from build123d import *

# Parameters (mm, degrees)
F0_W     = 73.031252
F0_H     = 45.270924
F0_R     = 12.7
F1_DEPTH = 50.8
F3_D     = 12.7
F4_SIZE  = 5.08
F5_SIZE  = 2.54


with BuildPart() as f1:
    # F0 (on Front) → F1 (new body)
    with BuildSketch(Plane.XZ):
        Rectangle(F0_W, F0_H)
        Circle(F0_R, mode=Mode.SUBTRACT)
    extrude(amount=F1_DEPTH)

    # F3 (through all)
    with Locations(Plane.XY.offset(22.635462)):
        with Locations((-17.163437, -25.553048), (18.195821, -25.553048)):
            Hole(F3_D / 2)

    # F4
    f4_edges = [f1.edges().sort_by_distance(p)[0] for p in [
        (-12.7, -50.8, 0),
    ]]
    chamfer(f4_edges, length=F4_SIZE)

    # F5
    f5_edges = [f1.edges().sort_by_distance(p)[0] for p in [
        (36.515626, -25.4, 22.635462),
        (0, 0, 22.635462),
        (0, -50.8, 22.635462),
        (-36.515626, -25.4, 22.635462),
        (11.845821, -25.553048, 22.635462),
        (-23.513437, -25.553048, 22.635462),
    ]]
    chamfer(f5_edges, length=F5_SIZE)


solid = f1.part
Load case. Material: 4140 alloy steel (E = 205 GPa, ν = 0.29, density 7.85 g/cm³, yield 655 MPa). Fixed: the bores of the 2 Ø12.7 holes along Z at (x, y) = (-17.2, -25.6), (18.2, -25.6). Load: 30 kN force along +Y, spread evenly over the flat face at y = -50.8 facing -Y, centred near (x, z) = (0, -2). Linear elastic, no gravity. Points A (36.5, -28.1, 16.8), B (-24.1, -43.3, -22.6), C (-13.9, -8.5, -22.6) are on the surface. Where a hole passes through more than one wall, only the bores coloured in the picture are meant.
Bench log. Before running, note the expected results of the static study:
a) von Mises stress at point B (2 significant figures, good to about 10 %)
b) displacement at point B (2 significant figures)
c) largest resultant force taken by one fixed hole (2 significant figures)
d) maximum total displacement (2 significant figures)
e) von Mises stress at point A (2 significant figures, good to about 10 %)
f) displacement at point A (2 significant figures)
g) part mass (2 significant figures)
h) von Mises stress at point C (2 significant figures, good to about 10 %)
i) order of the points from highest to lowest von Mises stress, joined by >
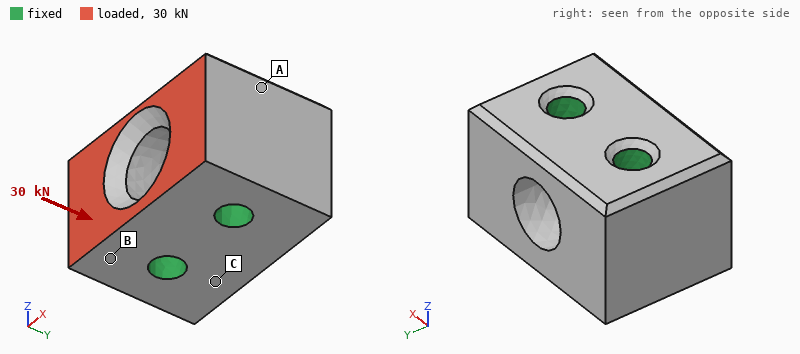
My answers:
16 MPa
1.7 µm
15 kN
3.2 µm
8.3 MPa
1.0 µm
1.0 kg
3.1 MPa
B > A > C
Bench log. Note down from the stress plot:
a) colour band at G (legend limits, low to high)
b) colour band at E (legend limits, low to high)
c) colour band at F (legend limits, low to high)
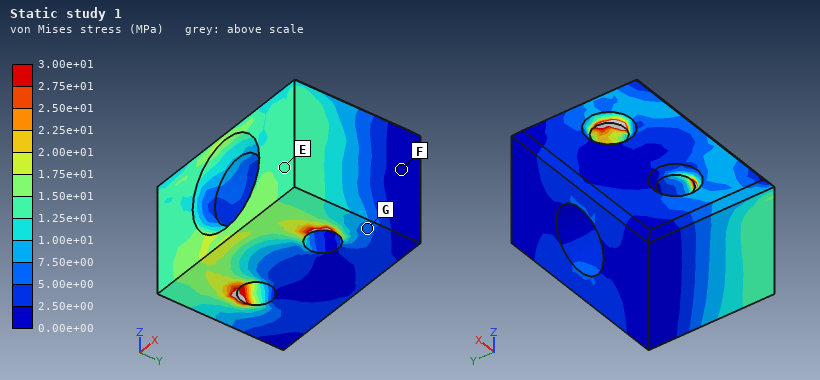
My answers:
5.00e+00 to 7.50e+00 MPa
1.25e+01 to 1.50e+01 MPa
0.00e+00 to 2.50e+00 MPa
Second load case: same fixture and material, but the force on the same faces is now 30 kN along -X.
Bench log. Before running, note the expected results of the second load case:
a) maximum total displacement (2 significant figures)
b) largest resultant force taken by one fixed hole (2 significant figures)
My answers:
9.8 µm
18 kN
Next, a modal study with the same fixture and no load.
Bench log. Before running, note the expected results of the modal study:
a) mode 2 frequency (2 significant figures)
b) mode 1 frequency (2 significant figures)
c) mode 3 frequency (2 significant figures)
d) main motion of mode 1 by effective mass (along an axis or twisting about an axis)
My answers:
24 kHz
21 kHz
25 kHz
twisting about Z
